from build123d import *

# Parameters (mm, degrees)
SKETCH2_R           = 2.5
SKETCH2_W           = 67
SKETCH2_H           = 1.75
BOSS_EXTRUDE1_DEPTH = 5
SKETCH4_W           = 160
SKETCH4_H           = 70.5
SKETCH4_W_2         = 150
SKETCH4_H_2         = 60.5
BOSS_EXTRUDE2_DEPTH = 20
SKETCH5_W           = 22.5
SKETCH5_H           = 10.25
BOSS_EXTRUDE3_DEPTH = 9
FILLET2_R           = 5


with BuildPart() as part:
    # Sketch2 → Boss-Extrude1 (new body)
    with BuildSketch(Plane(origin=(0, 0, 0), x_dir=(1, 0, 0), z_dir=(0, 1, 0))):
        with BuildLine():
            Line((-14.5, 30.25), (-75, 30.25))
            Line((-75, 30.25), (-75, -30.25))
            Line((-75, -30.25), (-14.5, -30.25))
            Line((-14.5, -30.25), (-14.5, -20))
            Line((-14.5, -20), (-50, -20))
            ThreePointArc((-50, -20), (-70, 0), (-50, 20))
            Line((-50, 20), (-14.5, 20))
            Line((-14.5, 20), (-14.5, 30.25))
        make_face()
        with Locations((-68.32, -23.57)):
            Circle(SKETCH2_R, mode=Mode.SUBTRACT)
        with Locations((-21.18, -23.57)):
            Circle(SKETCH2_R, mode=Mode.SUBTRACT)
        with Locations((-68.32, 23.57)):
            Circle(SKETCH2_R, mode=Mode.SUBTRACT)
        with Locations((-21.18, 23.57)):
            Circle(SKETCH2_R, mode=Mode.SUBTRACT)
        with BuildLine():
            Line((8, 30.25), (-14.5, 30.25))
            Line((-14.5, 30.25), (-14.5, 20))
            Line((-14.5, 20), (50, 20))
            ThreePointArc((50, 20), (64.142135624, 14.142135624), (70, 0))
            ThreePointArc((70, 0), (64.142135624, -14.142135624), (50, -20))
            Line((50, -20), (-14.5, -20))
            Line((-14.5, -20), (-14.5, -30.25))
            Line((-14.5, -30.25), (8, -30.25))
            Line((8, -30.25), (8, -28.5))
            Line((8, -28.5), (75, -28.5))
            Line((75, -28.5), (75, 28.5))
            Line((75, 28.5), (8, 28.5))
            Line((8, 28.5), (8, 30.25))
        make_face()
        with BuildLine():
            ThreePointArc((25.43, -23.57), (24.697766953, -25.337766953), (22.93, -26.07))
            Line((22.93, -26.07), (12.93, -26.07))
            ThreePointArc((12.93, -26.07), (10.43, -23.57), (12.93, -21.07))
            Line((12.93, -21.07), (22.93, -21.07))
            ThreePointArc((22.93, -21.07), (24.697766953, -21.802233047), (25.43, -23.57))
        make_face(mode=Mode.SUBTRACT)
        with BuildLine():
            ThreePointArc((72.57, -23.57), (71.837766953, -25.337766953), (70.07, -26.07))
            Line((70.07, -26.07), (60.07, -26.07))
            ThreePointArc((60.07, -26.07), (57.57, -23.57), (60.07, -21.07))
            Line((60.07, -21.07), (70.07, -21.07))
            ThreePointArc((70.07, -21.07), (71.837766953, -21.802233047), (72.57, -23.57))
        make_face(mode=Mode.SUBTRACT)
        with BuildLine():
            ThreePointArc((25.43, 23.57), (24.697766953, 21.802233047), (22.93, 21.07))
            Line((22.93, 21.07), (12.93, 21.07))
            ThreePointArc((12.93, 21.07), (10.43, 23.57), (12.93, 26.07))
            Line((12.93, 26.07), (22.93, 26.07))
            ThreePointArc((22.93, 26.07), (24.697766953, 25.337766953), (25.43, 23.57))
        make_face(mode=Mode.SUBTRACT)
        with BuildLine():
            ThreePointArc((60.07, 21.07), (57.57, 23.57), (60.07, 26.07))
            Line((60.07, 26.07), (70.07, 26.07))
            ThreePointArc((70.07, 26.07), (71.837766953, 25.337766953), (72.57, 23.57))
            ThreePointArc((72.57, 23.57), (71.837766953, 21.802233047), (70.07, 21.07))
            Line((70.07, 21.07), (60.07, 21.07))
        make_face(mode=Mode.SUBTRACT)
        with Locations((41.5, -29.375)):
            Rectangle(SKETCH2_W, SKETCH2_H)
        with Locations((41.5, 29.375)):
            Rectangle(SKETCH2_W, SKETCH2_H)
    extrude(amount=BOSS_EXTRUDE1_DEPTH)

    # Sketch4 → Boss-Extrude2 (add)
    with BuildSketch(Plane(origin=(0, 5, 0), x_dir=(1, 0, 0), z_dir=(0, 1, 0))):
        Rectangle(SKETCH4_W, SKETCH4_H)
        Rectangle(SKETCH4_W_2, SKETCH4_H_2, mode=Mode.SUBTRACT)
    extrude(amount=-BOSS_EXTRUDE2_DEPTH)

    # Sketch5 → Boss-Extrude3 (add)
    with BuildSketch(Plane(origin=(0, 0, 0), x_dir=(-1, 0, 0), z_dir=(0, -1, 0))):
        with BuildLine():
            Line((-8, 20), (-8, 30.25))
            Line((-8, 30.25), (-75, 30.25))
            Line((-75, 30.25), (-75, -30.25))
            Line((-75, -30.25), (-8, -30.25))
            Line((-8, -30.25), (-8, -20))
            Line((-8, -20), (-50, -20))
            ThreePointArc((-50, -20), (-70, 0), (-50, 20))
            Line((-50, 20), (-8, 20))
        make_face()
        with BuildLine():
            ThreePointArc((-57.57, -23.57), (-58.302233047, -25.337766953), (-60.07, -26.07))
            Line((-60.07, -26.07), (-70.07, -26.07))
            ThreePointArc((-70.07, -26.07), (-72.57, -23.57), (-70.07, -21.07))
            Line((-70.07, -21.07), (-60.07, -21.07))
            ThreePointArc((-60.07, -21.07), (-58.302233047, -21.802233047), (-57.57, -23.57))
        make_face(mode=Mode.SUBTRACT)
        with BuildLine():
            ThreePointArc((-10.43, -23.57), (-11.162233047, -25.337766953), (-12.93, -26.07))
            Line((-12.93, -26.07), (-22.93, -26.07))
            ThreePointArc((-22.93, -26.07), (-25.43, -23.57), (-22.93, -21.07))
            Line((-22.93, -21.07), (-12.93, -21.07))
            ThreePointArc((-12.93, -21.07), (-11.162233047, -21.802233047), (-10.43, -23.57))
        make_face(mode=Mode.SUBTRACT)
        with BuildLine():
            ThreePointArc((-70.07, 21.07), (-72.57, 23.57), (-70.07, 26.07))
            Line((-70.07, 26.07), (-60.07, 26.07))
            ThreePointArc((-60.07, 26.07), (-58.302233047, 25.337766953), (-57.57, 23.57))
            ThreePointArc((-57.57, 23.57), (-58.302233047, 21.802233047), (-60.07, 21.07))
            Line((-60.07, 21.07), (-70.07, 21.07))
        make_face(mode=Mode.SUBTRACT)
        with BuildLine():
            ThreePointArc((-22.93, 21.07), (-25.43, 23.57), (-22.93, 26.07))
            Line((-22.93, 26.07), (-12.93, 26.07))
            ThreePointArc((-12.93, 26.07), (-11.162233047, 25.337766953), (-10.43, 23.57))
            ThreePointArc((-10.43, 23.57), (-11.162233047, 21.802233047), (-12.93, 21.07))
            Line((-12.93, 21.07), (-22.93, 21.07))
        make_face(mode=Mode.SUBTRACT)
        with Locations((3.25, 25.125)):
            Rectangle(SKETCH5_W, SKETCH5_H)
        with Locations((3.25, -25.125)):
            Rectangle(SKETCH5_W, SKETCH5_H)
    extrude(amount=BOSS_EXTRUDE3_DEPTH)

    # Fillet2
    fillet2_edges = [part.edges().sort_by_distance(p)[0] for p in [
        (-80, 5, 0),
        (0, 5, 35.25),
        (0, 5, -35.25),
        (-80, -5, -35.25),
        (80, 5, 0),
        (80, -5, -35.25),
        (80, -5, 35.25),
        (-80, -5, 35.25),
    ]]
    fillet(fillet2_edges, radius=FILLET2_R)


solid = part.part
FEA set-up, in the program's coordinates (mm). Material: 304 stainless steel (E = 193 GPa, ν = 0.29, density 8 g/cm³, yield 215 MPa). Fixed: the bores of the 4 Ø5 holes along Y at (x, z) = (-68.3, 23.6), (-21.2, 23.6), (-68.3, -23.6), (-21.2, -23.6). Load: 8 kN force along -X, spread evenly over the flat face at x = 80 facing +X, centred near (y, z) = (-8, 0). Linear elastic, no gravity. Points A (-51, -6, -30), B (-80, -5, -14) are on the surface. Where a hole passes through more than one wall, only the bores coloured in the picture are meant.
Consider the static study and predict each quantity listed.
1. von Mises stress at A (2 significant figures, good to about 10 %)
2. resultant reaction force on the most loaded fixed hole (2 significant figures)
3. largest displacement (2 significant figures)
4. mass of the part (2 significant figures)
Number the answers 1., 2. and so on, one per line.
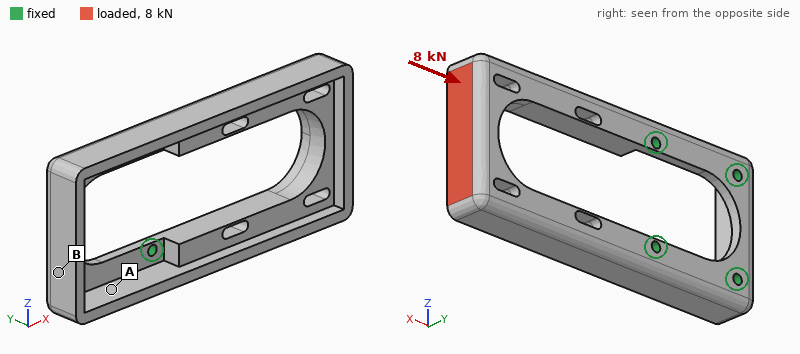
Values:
1. 25 MPa
2. 2.5 kN
3. 0.16 mm
4. 610 g
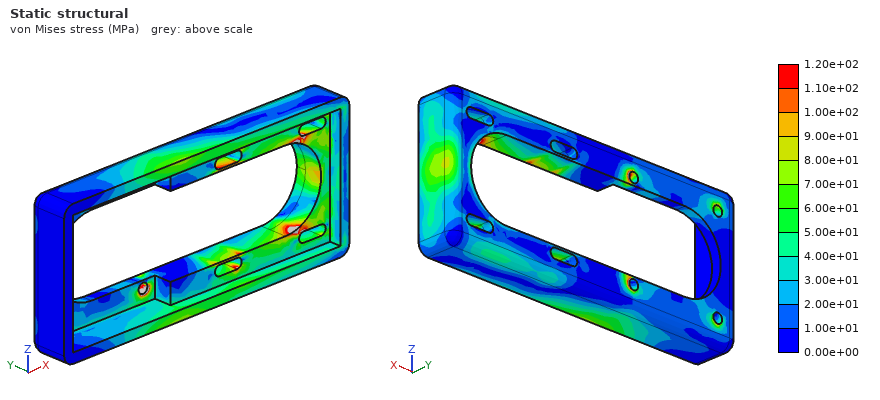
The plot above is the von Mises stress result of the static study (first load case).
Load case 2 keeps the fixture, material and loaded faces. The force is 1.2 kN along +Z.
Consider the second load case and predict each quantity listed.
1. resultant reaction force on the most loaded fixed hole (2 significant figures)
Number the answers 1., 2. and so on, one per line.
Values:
1. 1.1 kN
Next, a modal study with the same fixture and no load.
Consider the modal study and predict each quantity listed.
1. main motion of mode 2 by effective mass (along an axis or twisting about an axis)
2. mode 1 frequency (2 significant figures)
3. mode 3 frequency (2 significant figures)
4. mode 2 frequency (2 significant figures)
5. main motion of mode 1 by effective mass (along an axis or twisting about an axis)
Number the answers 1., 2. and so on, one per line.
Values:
1. along Z
2. 800 Hz
3. 1600 Hz
4. 1100 Hz
5. along Y
